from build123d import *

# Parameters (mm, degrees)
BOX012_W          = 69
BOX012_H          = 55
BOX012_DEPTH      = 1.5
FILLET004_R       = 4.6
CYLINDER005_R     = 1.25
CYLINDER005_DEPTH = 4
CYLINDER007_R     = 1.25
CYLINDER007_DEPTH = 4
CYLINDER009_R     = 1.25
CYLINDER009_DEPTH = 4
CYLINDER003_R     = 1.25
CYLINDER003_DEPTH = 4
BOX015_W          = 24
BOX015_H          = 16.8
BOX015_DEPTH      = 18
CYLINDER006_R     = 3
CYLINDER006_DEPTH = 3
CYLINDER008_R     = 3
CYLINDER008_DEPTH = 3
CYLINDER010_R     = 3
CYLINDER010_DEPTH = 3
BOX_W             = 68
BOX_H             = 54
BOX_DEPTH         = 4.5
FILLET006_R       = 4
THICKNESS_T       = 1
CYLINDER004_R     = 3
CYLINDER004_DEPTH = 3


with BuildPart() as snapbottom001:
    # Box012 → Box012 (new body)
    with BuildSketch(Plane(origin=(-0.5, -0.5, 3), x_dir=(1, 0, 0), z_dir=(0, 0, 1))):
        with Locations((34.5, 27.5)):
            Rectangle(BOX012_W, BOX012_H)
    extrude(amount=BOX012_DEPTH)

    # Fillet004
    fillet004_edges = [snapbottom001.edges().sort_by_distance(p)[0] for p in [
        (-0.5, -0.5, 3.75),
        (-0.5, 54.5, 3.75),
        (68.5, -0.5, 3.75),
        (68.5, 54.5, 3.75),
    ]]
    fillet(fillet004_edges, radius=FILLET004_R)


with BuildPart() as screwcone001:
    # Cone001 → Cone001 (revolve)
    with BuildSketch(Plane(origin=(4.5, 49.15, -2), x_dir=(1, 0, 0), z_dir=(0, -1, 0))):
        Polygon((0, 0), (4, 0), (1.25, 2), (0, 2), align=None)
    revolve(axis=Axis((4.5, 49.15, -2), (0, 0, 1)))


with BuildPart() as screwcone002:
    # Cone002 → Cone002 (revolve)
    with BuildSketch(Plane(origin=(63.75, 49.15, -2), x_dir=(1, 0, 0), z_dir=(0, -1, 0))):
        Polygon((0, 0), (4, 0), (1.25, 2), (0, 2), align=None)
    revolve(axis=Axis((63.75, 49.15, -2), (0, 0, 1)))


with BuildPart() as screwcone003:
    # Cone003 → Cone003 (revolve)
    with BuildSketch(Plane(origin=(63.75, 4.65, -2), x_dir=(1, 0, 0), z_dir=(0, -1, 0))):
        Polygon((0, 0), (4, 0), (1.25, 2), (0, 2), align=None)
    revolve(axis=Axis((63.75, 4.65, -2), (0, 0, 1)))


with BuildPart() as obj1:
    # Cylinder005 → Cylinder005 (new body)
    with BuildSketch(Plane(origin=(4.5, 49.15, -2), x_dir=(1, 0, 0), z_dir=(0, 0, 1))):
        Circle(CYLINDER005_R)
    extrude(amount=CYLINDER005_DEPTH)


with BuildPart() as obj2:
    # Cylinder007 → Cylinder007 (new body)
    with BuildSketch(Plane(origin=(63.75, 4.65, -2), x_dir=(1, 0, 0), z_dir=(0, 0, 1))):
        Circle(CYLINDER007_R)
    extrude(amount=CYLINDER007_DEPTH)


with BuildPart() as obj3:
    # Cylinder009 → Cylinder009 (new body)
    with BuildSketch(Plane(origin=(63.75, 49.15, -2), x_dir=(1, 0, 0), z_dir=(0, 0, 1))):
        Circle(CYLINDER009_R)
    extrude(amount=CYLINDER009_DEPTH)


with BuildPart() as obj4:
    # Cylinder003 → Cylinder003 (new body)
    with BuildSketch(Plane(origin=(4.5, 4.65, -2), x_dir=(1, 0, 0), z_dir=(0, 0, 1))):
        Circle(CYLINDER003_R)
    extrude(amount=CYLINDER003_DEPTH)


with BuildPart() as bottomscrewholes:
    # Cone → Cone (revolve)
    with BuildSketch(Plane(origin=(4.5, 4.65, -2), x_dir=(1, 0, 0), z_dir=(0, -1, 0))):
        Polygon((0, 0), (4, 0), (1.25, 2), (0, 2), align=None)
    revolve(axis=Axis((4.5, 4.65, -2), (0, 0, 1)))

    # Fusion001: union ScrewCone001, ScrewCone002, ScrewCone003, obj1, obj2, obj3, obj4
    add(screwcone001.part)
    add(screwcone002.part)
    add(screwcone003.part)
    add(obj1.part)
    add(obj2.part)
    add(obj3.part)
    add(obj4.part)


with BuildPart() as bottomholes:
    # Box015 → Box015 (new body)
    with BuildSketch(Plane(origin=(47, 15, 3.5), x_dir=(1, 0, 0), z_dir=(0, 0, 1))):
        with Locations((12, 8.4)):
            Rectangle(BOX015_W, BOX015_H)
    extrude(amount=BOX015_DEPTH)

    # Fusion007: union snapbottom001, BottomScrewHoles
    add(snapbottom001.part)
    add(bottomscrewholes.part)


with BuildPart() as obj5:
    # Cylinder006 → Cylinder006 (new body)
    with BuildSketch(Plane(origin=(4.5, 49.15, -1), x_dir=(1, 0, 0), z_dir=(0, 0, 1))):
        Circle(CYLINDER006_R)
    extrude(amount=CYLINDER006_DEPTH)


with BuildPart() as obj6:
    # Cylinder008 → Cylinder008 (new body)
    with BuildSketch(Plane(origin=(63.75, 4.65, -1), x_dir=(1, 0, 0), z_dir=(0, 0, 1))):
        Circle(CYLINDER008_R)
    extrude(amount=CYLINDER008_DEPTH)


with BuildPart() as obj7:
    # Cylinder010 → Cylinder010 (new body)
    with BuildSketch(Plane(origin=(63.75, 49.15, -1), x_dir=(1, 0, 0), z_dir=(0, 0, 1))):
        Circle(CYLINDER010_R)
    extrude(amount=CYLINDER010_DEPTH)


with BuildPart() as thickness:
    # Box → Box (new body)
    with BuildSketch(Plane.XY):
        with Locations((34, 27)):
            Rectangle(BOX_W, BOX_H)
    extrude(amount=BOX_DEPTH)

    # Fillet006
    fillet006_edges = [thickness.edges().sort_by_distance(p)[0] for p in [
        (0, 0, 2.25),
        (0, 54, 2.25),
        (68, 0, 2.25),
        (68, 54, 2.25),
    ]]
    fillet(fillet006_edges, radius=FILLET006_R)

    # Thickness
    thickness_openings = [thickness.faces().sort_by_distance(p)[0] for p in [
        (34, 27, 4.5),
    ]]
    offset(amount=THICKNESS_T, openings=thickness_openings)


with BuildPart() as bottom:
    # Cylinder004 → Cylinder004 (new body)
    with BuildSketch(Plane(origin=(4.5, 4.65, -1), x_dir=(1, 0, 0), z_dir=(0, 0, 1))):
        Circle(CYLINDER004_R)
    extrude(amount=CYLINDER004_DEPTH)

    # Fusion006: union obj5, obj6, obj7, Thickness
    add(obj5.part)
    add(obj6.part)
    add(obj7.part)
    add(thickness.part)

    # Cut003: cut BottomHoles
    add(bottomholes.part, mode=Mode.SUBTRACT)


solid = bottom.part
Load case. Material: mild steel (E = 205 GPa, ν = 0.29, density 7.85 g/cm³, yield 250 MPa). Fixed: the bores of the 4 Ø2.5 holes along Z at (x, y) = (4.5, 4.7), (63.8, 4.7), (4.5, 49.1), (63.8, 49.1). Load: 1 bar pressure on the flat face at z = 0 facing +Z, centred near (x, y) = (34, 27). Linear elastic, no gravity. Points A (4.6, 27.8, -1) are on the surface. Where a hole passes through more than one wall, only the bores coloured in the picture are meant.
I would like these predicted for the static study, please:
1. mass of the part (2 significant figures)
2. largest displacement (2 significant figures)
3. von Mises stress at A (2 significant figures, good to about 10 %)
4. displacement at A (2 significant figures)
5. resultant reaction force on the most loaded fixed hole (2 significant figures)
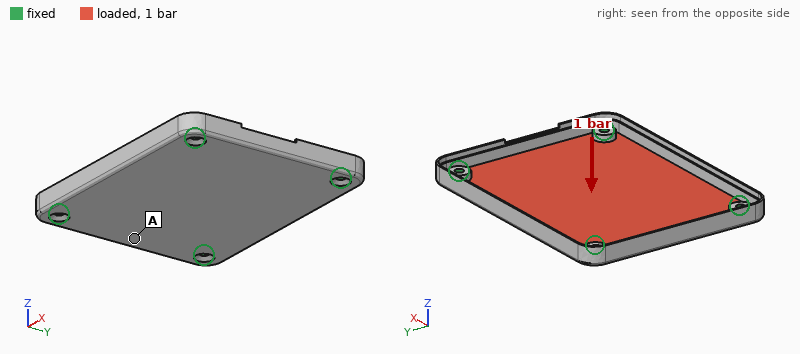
38 g
0.18 mm
29 MPa
0.036 mm
110 N
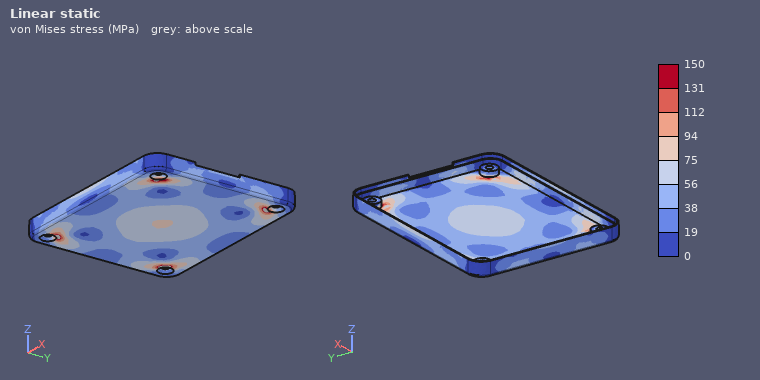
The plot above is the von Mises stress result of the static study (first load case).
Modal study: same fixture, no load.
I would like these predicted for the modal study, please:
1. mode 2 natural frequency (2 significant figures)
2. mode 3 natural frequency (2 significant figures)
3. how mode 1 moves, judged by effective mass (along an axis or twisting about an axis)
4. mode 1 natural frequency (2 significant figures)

3400 Hz
3500 Hz
along Z
1700 Hz
